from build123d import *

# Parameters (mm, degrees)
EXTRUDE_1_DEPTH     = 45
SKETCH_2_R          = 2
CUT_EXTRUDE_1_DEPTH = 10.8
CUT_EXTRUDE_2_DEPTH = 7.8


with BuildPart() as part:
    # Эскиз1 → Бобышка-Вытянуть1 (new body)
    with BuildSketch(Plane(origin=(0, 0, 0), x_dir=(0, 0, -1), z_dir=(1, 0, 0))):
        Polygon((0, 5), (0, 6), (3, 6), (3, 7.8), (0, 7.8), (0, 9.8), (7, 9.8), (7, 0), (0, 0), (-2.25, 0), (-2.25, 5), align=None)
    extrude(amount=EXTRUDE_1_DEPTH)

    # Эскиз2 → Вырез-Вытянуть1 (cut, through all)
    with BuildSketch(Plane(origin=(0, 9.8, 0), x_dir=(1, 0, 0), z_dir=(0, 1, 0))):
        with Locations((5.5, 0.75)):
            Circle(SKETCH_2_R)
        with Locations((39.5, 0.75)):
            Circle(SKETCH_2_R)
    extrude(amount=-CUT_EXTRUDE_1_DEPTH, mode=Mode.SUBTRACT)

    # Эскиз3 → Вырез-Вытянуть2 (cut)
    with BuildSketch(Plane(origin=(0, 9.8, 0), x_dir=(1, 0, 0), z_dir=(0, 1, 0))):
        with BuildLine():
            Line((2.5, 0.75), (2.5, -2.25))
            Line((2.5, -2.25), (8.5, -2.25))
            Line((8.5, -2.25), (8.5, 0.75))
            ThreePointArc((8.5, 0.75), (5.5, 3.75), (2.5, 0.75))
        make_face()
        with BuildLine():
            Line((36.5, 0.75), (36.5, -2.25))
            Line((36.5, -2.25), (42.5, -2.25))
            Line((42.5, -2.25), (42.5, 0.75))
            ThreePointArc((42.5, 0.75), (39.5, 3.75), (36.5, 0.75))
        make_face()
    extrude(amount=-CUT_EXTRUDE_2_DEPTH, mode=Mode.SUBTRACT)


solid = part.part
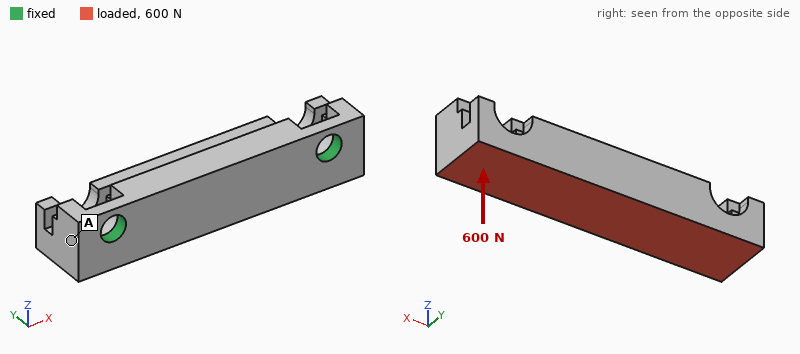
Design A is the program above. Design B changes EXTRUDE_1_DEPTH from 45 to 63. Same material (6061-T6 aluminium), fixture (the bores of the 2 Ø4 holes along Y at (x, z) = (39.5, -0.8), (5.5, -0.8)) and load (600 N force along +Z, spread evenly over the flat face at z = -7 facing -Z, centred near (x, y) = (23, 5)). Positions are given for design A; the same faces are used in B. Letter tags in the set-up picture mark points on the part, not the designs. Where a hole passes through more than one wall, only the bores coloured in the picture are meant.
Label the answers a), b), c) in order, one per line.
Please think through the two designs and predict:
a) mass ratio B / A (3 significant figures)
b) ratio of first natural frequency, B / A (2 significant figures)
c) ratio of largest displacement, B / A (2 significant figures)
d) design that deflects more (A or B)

a) 1.45
b) 0.52
c) 2.2
d) B
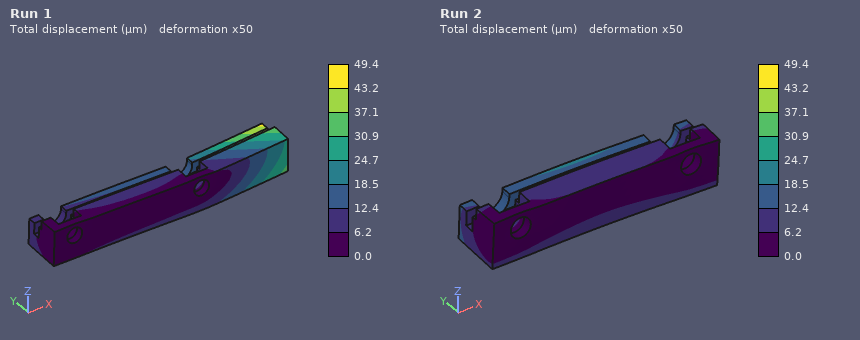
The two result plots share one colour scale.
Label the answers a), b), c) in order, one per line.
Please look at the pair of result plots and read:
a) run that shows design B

a) Run 1
